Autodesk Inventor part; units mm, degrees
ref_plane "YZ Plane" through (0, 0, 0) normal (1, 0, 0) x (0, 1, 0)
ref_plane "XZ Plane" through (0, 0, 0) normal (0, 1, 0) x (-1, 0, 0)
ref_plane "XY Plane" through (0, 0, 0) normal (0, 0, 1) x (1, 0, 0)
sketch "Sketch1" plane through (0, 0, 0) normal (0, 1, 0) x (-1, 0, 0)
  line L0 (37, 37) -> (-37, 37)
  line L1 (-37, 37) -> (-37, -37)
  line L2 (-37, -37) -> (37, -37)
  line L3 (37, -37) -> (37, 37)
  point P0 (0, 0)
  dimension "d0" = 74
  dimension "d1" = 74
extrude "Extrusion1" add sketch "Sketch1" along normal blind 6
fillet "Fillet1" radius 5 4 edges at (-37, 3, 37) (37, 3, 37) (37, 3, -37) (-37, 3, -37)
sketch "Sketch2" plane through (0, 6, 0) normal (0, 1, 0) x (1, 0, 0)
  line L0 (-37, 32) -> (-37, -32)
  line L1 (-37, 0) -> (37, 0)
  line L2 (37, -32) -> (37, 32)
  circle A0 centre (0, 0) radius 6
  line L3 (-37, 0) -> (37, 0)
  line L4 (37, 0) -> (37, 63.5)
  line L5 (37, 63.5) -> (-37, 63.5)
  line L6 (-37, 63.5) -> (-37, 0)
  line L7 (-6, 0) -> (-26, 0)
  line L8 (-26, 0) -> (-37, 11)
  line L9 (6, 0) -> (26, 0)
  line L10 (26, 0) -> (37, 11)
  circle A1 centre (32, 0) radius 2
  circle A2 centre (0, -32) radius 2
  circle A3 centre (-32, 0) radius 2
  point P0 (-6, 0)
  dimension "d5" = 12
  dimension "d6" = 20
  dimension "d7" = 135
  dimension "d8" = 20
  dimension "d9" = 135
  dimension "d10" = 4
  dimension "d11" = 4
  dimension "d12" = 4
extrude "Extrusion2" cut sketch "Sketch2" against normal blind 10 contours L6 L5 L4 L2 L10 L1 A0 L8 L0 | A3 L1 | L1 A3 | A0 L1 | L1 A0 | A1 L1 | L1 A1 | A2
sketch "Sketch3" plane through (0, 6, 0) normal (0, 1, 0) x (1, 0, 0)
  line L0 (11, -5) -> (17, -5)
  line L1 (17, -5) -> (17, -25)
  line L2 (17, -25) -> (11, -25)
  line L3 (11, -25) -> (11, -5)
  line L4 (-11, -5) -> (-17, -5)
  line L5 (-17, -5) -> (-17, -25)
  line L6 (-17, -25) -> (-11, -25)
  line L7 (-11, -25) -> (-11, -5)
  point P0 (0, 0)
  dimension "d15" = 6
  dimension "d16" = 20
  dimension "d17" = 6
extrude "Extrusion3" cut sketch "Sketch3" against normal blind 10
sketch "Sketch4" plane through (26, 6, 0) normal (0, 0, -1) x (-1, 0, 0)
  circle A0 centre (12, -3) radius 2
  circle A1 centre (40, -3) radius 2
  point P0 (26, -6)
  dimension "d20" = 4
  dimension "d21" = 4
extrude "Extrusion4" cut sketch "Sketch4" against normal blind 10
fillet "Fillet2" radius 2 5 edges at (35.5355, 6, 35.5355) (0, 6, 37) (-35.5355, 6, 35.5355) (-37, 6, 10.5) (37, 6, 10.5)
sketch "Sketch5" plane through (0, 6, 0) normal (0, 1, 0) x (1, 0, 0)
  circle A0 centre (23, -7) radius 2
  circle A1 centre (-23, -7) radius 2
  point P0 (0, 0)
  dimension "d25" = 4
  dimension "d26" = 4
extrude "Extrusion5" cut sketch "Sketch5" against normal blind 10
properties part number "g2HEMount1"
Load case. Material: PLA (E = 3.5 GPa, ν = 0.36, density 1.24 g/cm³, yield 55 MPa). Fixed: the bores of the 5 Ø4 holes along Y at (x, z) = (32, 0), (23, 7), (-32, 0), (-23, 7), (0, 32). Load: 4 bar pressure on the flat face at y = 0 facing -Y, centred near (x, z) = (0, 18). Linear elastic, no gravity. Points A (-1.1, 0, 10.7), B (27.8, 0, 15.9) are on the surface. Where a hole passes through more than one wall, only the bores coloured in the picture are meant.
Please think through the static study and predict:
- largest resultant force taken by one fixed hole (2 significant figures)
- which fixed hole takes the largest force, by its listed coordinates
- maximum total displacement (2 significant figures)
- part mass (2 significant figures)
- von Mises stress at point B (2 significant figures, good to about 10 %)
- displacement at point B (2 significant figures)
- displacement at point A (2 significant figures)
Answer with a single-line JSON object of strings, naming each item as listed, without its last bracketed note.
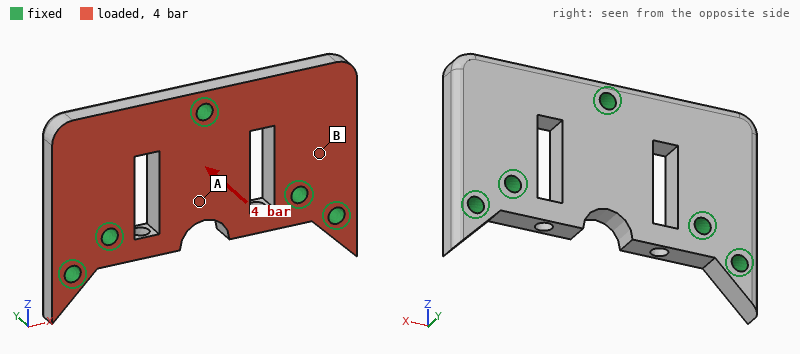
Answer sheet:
{"largest resultant force taken by one fixed hole": "380 N", "which fixed hole takes the largest force, by its listed coordinates": "(0, 32)", "maximum total displacement": "0.38 mm", "part mass": "18 g", "von Mises stress at point B": "6.3 MPa", "displacement at point B": "0.086 mm", "displacement at point A": "0.089 mm"}
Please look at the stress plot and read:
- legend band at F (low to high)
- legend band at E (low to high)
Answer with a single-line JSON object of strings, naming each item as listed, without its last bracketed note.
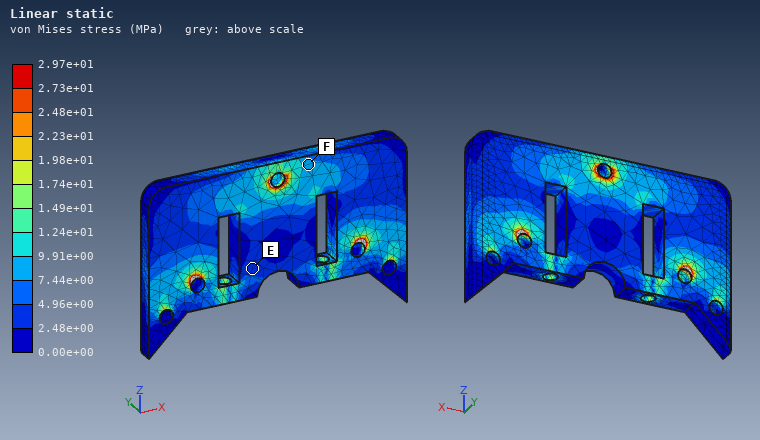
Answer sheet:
{"legend band at F": "7.44e+00 to 9.91e+00 MPa", "legend band at E": "2.48e+00 to 4.96e+00 MPa"}
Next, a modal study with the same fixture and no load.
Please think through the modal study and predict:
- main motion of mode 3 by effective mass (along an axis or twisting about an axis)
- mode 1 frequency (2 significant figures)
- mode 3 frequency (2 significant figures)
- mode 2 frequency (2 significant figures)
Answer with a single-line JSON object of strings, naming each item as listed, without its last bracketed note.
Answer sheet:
{"main motion of mode 3 by effective mass": "along Y", "mode 1 frequency": "2500 Hz", "mode 3 frequency": "3900 Hz", "mode 2 frequency": "2600 Hz"}
